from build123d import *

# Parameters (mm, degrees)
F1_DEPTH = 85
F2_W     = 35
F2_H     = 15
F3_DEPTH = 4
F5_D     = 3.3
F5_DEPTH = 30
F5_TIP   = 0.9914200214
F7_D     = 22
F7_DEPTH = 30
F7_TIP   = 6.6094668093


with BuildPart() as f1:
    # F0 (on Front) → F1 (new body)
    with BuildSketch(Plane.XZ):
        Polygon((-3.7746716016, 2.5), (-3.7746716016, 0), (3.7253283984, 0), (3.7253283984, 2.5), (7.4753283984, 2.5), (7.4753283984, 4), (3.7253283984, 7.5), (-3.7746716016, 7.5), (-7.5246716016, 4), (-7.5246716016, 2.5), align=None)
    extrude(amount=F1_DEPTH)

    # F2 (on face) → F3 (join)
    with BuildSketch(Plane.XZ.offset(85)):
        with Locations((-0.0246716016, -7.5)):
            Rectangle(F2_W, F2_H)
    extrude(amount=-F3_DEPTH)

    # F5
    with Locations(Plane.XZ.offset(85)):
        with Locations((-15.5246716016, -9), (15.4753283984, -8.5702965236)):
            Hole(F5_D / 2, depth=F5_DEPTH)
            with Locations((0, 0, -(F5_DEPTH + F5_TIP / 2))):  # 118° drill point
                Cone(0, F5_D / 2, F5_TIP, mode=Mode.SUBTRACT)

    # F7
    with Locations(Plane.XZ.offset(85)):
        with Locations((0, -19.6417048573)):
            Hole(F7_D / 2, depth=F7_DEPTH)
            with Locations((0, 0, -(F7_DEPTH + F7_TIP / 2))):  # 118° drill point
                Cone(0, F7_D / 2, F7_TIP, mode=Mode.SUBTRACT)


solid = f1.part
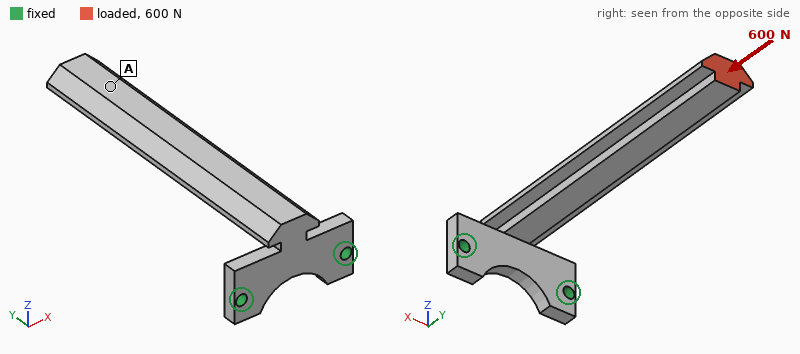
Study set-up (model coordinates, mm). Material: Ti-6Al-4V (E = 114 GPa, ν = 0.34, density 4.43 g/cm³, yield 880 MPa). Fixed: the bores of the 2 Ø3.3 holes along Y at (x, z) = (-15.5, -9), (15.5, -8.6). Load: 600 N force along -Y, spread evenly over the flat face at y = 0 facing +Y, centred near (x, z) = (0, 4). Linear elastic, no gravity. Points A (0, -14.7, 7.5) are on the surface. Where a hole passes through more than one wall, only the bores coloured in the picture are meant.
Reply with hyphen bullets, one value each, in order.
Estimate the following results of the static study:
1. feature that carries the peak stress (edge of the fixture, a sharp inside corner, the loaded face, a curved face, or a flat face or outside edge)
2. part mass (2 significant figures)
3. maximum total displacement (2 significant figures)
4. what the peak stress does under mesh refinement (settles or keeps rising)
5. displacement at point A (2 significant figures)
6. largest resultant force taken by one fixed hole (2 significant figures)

- edge of the fixture
- 38 g
- 0.68 mm
- keeps rising
- 0.56 mm
- 300 N
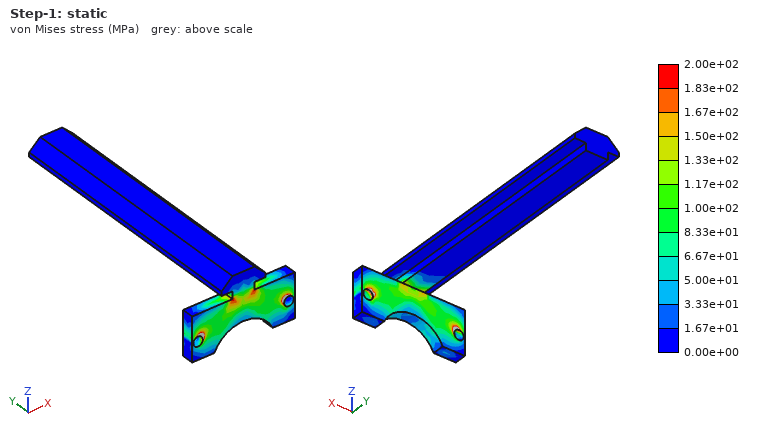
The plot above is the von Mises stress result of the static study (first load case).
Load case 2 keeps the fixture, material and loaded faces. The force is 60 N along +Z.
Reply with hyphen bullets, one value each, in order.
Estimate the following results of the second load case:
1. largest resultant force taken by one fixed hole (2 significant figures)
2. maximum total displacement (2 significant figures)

- 44 N
- 1.1 mm
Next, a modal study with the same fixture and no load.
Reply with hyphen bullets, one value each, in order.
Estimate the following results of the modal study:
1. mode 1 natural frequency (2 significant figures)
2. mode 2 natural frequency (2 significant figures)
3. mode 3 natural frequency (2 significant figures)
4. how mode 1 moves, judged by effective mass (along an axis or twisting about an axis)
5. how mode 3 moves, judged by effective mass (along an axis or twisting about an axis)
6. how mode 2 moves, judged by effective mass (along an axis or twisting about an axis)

- 400 Hz
- 630 Hz
- 3000 Hz
- along Z
- along Y
- along X
